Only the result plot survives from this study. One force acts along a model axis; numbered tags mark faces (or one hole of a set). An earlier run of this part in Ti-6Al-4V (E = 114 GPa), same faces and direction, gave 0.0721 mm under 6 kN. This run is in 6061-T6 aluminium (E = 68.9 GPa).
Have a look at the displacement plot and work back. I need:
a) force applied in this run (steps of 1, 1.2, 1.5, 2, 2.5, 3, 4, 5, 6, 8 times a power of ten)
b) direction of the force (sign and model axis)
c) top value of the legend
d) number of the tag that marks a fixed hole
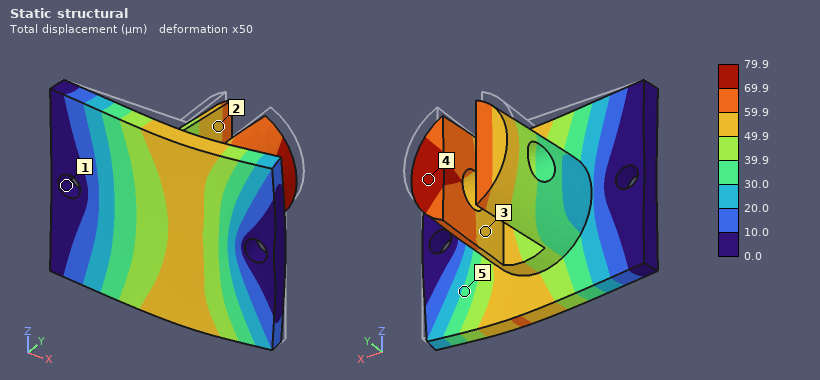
4 kN
-Y
79.9 µm
1
